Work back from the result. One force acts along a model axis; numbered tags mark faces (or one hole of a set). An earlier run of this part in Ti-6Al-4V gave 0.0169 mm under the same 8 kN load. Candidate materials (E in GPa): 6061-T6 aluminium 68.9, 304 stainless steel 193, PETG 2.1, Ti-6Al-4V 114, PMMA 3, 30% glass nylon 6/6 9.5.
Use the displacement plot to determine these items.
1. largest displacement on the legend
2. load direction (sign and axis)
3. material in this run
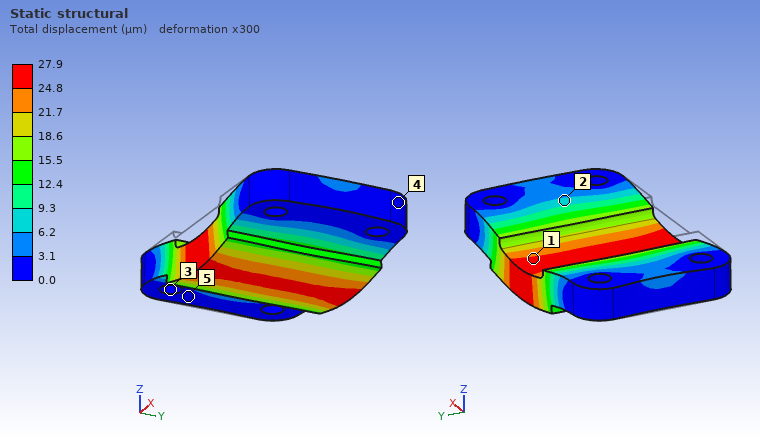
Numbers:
27.9 µm
-Z
6061-T6 aluminium
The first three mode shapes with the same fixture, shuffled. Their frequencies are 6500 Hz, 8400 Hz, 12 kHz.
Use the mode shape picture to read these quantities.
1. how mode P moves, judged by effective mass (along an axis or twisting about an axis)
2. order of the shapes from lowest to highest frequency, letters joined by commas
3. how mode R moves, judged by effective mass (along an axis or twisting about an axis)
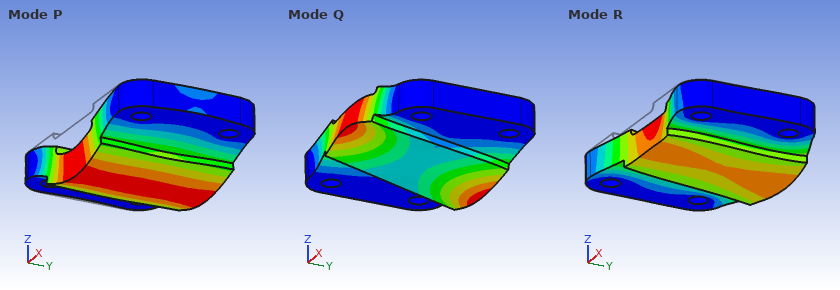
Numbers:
along Z
P, Q, R
along Y
